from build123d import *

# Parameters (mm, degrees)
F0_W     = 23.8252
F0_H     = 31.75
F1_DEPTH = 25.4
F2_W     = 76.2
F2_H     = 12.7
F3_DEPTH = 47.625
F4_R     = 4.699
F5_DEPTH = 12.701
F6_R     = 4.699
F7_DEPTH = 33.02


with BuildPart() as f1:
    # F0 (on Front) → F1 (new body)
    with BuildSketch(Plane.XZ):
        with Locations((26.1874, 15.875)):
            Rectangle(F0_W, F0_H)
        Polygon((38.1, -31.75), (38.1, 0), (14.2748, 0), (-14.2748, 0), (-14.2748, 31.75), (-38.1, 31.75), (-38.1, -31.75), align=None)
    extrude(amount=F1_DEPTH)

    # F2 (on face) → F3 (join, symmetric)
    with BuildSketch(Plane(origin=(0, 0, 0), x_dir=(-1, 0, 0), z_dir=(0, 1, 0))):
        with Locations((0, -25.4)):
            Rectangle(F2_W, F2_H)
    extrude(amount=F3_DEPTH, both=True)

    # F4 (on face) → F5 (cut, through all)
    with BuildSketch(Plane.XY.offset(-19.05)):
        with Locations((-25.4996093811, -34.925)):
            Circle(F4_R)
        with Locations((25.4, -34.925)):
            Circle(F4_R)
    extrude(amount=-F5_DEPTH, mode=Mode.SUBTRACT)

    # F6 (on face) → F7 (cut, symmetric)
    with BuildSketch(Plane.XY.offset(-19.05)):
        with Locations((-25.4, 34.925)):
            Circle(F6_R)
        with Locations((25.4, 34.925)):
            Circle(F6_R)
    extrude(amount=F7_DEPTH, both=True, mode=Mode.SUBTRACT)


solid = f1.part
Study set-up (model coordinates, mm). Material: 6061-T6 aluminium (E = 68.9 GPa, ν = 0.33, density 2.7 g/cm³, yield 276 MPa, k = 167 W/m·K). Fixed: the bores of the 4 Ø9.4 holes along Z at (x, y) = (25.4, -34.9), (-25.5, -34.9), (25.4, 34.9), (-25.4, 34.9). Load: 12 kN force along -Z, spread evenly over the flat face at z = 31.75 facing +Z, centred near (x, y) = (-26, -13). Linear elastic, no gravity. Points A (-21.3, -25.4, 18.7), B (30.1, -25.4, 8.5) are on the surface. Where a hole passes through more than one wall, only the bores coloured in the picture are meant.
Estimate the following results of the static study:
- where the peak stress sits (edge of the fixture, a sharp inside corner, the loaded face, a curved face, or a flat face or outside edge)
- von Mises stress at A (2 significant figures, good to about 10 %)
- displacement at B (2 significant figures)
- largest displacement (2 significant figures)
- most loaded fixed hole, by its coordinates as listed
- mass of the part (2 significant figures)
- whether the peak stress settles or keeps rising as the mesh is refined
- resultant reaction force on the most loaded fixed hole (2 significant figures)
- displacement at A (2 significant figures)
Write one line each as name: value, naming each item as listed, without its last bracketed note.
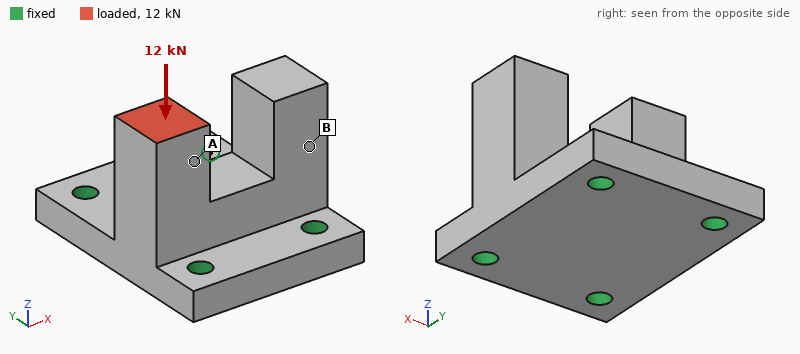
where the peak stress sits: edge of the fixture
von Mises stress at A: 20 MPa
displacement at B: 17 µm
largest displacement: 79 µm
most loaded fixed hole, by its coordinates as listed: (-25.5, -34.9)
mass of the part: 440 g
whether the peak stress settles or keeps rising as the mesh is refined: keeps rising
resultant reaction force on the most loaded fixed hole: 8.9 kN
displacement at A: 47 µm
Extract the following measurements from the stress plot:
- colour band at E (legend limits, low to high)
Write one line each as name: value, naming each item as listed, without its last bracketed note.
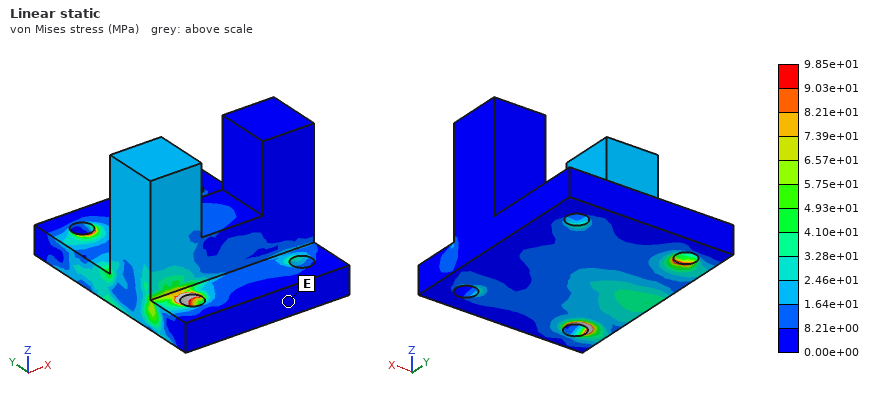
colour band at E: 0.00e+00 to 8.21e+00 MPa
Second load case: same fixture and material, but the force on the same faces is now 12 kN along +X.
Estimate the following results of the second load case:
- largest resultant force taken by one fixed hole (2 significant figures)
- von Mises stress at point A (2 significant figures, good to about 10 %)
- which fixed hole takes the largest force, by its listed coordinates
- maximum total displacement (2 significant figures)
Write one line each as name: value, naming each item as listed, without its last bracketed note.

largest resultant force taken by one fixed hole: 12 kN
von Mises stress at point A: 57 MPa
which fixed hole takes the largest force, by its listed coordinates: (25.4, -34.9)
maximum total displacement: 0.32 mm
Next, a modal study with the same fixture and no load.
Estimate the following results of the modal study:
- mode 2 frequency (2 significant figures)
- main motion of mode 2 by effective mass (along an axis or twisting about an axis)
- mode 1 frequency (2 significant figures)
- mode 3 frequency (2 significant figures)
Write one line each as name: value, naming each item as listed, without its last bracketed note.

mode 2 frequency: 5000 Hz
main motion of mode 2 by effective mass: along X
mode 1 frequency: 4400 Hz
mode 3 frequency: 6300 Hz
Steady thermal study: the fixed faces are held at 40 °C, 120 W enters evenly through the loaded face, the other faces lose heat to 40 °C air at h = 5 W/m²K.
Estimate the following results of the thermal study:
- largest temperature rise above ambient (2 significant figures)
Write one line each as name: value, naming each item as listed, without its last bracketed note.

largest temperature rise above ambient: 67 K
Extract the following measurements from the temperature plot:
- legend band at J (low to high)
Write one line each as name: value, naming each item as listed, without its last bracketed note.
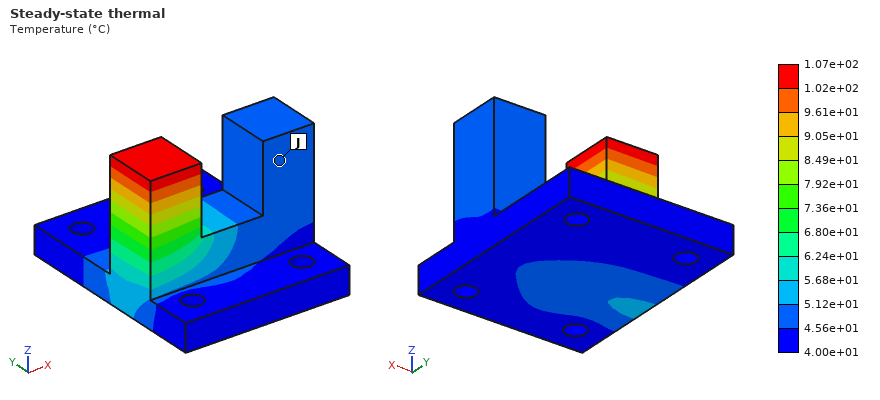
legend band at J: 4.56e+01 to 5.12e+01 °C
